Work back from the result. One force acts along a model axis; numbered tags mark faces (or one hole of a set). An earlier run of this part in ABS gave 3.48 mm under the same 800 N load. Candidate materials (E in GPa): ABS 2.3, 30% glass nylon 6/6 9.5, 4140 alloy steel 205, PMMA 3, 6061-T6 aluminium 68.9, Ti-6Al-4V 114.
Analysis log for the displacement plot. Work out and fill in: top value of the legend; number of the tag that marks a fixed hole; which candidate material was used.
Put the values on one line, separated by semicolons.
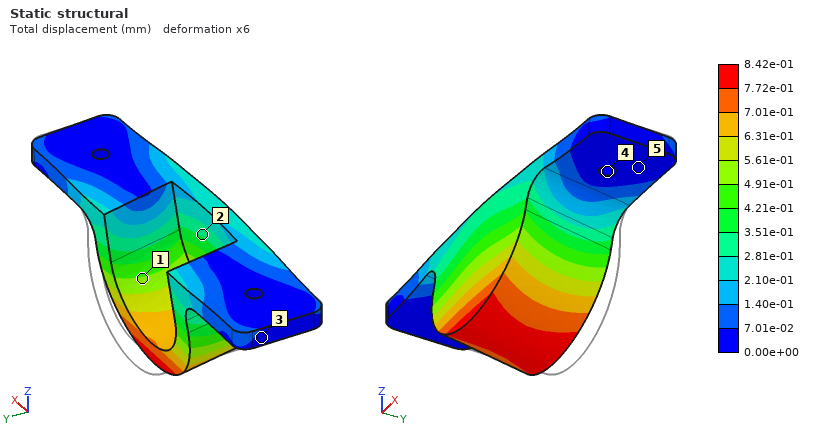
8.42e-01 mm; 4; 30% glass nylon 6/6
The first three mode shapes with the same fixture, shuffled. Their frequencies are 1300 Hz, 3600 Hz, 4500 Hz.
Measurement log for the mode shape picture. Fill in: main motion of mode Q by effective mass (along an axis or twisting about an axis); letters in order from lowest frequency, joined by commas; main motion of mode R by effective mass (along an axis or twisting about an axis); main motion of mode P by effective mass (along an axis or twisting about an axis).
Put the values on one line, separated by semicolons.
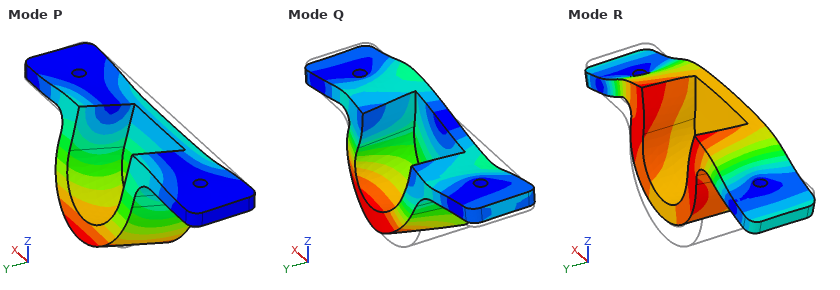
along X; P, R, Q; along Z; along Y
